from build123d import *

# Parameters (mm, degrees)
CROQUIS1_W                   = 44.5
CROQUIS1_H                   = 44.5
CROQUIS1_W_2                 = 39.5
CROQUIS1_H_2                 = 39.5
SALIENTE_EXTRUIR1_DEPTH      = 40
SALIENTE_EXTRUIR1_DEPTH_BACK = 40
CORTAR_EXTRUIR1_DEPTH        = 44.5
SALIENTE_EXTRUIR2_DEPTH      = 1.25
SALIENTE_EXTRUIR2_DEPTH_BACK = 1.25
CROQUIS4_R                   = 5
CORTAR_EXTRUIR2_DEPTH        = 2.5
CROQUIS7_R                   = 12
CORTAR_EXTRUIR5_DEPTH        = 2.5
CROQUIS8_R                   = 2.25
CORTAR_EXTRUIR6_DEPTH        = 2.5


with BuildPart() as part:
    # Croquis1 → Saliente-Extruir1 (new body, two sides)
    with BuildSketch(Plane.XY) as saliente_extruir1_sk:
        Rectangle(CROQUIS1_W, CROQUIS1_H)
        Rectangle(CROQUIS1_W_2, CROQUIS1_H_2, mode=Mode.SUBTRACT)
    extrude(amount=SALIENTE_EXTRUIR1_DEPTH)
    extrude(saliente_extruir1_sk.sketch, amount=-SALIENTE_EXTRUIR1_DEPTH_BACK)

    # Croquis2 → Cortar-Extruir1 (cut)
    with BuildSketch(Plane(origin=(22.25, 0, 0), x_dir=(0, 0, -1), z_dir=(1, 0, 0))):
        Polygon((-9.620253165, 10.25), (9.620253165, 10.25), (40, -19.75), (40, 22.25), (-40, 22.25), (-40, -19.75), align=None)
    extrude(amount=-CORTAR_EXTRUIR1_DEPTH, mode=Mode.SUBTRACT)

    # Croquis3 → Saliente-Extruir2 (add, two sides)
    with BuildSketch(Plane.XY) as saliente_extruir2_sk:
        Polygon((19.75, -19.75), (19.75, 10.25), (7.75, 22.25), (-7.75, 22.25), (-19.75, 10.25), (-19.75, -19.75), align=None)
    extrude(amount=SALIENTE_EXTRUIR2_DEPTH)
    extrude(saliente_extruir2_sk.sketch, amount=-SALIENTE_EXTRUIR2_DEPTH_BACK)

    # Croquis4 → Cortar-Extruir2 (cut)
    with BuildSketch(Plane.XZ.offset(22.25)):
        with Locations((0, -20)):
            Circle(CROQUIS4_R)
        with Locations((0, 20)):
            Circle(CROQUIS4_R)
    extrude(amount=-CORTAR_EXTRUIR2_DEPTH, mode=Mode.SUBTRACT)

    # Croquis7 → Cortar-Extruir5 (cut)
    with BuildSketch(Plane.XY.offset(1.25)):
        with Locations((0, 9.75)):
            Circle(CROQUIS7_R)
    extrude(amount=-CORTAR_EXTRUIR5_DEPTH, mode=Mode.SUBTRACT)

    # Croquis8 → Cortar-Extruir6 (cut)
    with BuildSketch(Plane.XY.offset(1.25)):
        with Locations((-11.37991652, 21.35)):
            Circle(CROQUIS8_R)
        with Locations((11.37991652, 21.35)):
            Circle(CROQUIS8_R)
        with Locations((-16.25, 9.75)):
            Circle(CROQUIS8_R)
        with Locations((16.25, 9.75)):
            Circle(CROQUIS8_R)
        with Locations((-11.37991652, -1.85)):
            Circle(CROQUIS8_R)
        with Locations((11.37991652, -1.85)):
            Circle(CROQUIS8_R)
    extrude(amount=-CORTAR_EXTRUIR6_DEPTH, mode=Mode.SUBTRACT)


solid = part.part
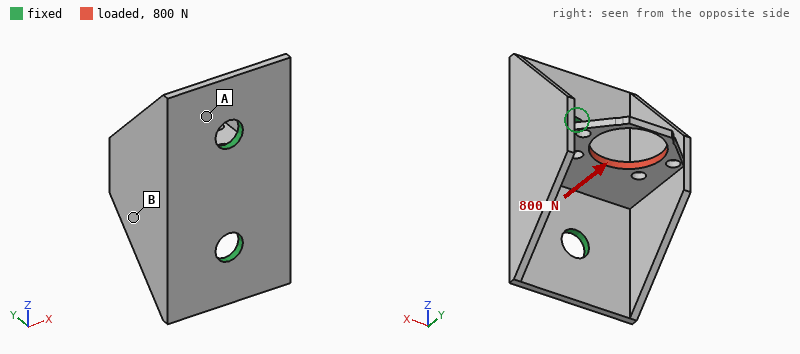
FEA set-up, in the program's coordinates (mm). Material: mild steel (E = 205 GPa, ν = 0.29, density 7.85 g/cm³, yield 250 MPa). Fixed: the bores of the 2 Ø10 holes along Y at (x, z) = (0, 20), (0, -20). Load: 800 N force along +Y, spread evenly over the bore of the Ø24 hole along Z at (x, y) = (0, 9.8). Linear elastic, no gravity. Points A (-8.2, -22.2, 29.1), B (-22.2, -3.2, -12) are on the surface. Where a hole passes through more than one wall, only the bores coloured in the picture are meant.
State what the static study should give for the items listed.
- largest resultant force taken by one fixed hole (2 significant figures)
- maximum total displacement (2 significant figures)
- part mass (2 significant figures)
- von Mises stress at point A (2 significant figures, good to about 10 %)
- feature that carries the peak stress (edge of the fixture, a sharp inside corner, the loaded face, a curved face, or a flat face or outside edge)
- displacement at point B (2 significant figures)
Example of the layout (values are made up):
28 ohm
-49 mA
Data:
410 N
32 µm
140 g
17 MPa
a flat face or outside edge
12 µm
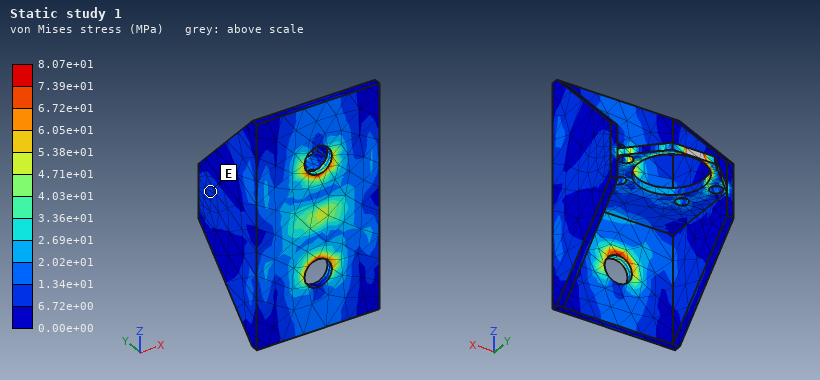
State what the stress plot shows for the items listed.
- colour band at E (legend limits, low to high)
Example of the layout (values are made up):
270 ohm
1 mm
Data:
6.72e+00 to 1.34e+01 MPa
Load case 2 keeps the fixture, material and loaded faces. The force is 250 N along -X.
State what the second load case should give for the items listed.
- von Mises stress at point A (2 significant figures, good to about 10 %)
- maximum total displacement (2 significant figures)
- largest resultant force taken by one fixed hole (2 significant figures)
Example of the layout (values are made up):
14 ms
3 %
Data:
21 MPa
46 µm
130 N
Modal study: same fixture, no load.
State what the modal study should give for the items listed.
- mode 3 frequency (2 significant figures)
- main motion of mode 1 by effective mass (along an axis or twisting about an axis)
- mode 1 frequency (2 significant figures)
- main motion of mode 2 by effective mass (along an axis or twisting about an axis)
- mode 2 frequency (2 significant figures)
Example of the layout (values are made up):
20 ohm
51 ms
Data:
3200 Hz
along X
2000 Hz
along Z
2900 Hz
